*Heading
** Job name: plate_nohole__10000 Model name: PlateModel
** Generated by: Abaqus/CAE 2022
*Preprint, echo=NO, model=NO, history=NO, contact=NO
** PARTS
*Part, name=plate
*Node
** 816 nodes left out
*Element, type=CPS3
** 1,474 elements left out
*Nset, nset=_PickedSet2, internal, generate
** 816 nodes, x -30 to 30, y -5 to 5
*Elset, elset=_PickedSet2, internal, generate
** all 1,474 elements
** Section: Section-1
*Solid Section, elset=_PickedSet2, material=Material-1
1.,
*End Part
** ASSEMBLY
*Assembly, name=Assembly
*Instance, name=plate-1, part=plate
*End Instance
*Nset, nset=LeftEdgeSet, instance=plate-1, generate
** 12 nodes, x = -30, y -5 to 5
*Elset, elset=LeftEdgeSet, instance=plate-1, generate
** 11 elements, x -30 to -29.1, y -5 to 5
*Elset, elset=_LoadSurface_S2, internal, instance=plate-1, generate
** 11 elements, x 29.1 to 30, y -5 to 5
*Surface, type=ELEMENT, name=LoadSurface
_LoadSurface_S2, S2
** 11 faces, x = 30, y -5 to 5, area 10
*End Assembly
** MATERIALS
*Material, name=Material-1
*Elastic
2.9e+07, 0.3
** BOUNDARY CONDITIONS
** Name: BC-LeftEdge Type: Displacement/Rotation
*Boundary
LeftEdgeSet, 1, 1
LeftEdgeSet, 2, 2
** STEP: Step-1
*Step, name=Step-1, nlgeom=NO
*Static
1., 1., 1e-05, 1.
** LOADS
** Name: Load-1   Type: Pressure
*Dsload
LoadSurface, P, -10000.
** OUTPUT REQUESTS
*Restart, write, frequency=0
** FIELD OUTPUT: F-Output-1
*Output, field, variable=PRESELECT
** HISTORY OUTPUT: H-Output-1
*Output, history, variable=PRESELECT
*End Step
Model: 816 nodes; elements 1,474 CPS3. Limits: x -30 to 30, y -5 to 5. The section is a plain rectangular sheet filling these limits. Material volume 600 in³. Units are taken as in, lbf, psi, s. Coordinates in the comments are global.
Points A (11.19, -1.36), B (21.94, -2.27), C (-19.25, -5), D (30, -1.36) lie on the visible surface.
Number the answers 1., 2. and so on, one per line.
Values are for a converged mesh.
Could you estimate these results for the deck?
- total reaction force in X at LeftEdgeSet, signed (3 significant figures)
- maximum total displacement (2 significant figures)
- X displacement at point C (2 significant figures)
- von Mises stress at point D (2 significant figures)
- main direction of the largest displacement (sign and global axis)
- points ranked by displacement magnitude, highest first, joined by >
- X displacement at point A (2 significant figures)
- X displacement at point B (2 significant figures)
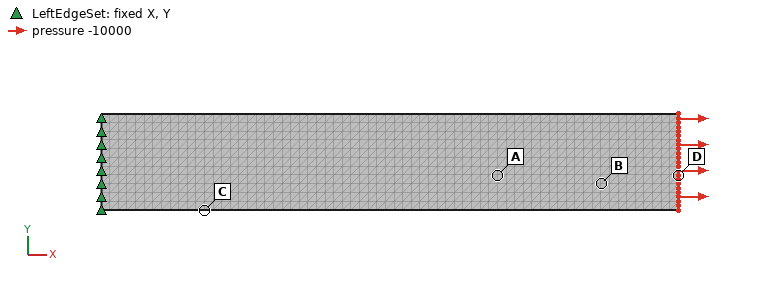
1. -1.00e+05 lbf
2. 0.021 in
3. 0.0037 in
4. 10000 psi
5. +X
6. D > B > A > C
7. 0.014 in
8. 0.018 in
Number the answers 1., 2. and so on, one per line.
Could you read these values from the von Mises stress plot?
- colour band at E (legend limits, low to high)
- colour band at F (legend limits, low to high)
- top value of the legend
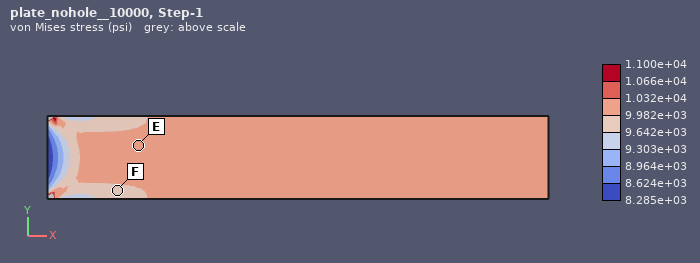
1. 9.982e+03 to 1.032e+04 psi
2. 9.642e+03 to 9.982e+03 psi
3. 1.100e+04 psi
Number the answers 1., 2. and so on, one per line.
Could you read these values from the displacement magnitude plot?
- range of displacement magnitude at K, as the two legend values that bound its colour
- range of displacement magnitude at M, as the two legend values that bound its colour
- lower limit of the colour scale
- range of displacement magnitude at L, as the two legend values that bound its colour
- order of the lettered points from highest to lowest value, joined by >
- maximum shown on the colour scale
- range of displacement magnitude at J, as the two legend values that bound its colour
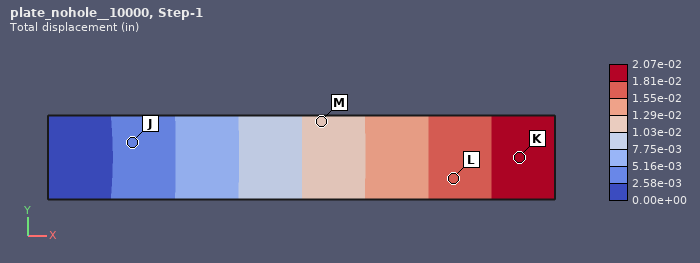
1. 1.81e-02 to 2.07e-02 in
2. 1.03e-02 to 1.29e-02 in
3. 0.00e+00 in
4. 1.55e-02 to 1.81e-02 in
5. K > L > M > J
6. 2.07e-02 in
7. 2.58e-03 to 5.16e-03 in
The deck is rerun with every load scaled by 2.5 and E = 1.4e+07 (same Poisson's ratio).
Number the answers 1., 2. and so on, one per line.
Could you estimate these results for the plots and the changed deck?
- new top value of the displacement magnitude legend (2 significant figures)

1. 0.11 in
